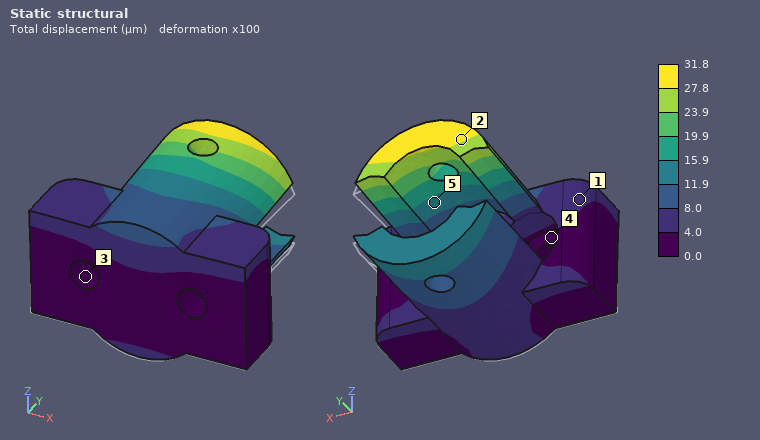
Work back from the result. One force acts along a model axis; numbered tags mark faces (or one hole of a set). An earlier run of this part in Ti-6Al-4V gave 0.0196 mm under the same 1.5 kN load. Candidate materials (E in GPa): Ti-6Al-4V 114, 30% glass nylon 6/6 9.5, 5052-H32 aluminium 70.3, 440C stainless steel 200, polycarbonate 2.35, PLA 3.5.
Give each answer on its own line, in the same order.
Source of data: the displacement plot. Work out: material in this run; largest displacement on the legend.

5052-H32 aluminium
31.8 µm
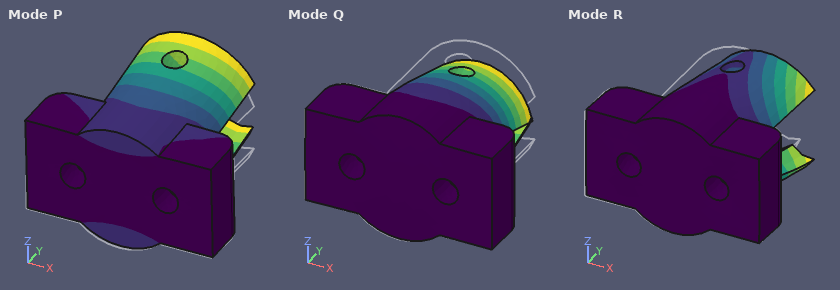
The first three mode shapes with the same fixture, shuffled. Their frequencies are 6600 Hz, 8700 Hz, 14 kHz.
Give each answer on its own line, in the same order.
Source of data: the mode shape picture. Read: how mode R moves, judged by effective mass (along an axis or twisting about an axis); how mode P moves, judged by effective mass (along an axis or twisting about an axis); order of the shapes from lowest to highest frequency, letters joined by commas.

along X
along Z
P, Q, R
